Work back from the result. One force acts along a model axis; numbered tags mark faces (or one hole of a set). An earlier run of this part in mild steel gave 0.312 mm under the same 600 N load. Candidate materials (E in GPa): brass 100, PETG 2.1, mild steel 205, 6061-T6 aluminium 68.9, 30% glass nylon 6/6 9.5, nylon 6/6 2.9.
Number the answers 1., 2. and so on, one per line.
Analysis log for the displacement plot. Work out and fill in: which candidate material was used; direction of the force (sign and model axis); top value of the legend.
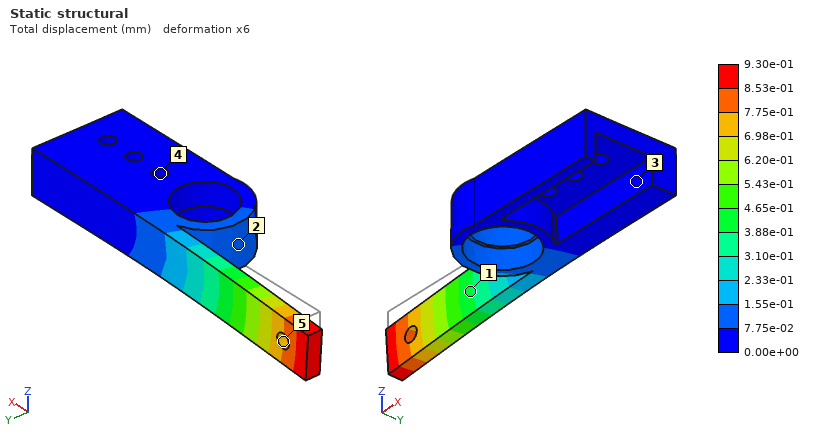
1. 6061-T6 aluminium
2. -Z
3. 9.30e-01 mm
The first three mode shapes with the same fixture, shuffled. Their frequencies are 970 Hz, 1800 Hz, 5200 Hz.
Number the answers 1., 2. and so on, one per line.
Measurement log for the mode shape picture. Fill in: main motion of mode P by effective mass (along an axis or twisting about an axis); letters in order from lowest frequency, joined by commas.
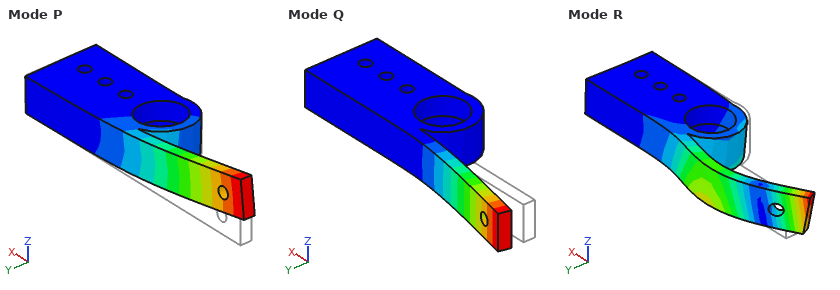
1. along Z
2. Q, P, R
